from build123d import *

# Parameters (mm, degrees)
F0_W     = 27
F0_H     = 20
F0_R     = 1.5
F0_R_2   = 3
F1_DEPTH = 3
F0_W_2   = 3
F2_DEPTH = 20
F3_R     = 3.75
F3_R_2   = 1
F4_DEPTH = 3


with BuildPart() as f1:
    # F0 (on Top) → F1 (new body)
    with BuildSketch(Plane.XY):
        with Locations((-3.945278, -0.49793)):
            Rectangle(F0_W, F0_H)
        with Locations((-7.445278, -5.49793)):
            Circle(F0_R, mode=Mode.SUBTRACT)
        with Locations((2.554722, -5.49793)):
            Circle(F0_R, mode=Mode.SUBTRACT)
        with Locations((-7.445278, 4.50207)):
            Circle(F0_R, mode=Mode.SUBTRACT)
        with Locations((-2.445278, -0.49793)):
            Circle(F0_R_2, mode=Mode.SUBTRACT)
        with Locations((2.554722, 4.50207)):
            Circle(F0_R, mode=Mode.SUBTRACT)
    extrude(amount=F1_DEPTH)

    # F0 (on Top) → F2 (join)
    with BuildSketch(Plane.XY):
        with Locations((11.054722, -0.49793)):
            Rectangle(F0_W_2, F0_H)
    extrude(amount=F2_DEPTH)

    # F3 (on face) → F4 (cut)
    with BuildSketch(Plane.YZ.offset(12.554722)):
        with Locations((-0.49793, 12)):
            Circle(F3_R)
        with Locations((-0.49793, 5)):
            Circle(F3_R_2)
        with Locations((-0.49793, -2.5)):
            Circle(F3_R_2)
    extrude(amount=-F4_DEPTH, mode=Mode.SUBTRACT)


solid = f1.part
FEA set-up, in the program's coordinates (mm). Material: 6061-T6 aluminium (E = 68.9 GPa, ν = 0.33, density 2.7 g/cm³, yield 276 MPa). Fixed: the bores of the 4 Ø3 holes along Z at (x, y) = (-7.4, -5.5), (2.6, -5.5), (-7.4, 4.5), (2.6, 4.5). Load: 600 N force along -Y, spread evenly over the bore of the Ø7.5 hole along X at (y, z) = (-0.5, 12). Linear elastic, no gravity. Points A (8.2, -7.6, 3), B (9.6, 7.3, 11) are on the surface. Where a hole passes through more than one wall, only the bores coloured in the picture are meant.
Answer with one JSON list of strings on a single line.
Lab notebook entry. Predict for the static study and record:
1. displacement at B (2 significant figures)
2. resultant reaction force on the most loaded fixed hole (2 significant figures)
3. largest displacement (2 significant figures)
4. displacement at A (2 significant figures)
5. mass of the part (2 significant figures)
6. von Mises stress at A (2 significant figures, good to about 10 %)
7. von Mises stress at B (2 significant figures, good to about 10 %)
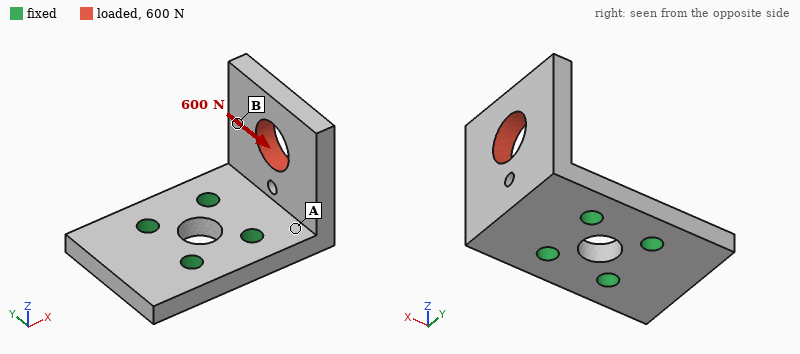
["0.065 mm", "670 N", "0.11 mm", "0.021 mm", "6.8 g", "87 MPa", "34 MPa"]
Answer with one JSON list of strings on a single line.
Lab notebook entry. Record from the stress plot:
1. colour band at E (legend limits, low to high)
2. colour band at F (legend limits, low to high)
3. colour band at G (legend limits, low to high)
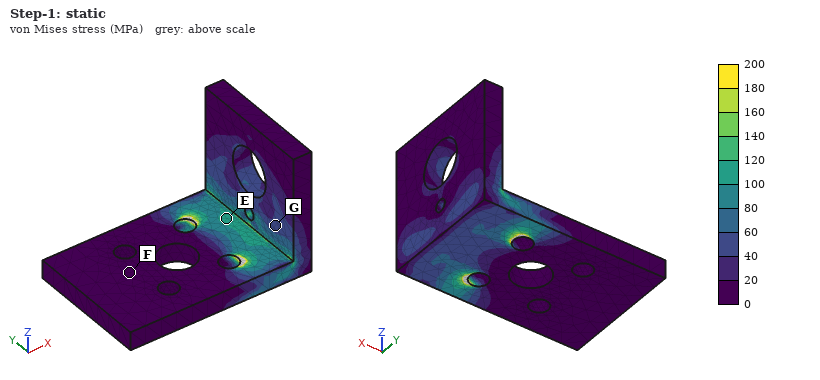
["100 to 120 MPa", "0 to 20 MPa", "40 to 60 MPa"]
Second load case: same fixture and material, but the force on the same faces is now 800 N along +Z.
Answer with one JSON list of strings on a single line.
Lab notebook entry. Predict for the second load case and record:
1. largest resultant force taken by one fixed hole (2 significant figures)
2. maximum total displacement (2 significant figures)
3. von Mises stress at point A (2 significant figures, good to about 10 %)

["440 N", "0.16 mm", "70 MPa"]
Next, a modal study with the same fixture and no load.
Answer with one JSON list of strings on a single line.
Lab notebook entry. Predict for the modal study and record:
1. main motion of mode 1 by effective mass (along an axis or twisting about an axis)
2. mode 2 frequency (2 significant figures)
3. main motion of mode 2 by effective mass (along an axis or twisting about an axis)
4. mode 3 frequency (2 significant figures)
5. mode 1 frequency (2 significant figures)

["along X", "8600 Hz", "along Y", "13 kHz", "4500 Hz"]
